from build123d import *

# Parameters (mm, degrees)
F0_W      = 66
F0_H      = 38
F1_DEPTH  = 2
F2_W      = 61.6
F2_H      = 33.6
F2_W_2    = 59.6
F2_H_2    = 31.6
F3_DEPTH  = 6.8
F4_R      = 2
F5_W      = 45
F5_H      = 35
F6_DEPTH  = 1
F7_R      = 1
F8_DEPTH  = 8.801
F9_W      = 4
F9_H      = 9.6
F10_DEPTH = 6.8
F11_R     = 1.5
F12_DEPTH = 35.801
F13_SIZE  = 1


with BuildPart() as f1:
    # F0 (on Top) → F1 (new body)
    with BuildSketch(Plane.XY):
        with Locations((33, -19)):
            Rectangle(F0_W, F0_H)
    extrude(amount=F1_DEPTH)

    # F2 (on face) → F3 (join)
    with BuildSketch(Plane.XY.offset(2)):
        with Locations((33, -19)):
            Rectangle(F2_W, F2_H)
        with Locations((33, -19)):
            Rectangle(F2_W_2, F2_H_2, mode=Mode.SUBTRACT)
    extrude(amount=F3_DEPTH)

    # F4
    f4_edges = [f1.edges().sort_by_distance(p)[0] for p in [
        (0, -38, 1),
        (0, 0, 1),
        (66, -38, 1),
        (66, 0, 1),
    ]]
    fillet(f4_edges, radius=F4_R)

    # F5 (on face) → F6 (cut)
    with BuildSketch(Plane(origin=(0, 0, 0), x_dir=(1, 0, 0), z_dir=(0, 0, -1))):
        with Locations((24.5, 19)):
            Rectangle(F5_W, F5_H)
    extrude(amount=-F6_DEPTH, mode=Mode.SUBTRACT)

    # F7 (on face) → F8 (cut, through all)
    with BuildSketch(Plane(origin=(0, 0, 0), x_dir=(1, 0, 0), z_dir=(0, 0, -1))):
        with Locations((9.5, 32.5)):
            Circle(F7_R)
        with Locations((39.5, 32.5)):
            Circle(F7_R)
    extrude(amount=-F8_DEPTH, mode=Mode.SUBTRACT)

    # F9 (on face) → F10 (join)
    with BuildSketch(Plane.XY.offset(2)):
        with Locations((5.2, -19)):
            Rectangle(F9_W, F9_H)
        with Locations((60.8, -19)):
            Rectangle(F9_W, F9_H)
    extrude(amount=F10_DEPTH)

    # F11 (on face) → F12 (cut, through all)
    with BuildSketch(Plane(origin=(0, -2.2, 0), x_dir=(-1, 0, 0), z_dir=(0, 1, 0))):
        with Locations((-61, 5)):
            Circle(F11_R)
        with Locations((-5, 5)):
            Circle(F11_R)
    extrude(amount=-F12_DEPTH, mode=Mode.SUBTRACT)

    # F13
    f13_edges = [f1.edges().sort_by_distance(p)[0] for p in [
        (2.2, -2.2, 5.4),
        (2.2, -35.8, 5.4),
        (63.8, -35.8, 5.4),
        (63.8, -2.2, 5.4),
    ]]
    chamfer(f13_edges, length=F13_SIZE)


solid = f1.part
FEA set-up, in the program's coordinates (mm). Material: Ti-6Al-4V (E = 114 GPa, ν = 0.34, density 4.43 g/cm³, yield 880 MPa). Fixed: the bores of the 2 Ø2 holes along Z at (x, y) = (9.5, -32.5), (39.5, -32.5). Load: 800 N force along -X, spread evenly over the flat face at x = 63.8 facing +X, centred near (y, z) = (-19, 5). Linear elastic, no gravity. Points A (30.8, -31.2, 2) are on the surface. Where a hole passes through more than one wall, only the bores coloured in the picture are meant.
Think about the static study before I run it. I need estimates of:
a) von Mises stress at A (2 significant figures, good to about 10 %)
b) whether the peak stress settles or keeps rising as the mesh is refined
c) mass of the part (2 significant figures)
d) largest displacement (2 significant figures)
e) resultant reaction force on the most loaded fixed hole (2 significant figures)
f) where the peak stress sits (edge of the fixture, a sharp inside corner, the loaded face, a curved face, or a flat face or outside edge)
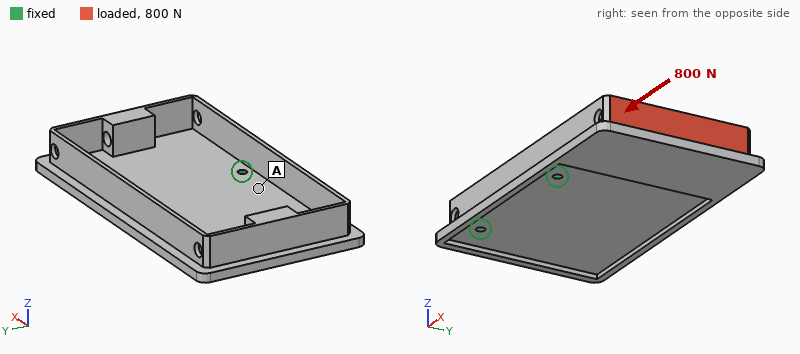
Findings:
22 MPa
keeps rising
22 g
0.52 mm
540 N
edge of the fixture
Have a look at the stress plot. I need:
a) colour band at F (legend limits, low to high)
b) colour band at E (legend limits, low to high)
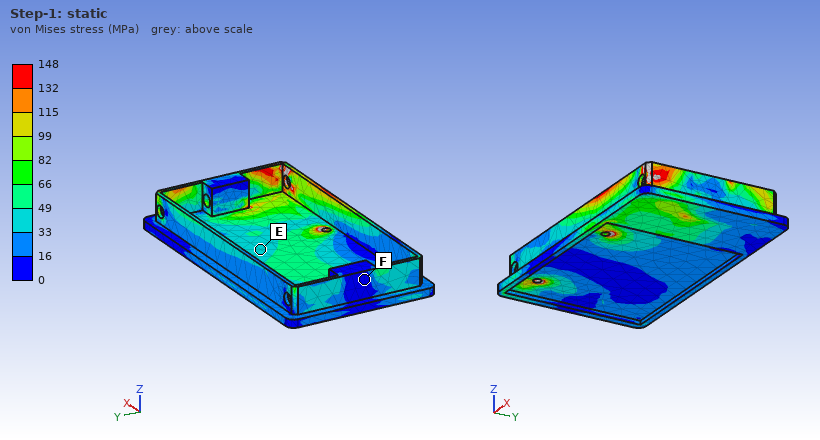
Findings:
0 to 16 MPa
33 to 49 MPa
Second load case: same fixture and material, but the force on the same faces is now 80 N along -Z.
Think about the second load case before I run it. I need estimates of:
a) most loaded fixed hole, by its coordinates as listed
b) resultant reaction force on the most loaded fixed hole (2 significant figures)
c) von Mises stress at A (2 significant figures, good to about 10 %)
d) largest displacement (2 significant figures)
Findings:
(39.5, -32.5)
160 N
34 MPa
0.76 mm
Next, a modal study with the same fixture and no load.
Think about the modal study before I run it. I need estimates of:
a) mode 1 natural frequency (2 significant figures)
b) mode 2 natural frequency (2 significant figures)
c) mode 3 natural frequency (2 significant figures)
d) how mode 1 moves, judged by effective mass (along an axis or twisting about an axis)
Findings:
590 Hz
1200 Hz
3800 Hz
along Z
